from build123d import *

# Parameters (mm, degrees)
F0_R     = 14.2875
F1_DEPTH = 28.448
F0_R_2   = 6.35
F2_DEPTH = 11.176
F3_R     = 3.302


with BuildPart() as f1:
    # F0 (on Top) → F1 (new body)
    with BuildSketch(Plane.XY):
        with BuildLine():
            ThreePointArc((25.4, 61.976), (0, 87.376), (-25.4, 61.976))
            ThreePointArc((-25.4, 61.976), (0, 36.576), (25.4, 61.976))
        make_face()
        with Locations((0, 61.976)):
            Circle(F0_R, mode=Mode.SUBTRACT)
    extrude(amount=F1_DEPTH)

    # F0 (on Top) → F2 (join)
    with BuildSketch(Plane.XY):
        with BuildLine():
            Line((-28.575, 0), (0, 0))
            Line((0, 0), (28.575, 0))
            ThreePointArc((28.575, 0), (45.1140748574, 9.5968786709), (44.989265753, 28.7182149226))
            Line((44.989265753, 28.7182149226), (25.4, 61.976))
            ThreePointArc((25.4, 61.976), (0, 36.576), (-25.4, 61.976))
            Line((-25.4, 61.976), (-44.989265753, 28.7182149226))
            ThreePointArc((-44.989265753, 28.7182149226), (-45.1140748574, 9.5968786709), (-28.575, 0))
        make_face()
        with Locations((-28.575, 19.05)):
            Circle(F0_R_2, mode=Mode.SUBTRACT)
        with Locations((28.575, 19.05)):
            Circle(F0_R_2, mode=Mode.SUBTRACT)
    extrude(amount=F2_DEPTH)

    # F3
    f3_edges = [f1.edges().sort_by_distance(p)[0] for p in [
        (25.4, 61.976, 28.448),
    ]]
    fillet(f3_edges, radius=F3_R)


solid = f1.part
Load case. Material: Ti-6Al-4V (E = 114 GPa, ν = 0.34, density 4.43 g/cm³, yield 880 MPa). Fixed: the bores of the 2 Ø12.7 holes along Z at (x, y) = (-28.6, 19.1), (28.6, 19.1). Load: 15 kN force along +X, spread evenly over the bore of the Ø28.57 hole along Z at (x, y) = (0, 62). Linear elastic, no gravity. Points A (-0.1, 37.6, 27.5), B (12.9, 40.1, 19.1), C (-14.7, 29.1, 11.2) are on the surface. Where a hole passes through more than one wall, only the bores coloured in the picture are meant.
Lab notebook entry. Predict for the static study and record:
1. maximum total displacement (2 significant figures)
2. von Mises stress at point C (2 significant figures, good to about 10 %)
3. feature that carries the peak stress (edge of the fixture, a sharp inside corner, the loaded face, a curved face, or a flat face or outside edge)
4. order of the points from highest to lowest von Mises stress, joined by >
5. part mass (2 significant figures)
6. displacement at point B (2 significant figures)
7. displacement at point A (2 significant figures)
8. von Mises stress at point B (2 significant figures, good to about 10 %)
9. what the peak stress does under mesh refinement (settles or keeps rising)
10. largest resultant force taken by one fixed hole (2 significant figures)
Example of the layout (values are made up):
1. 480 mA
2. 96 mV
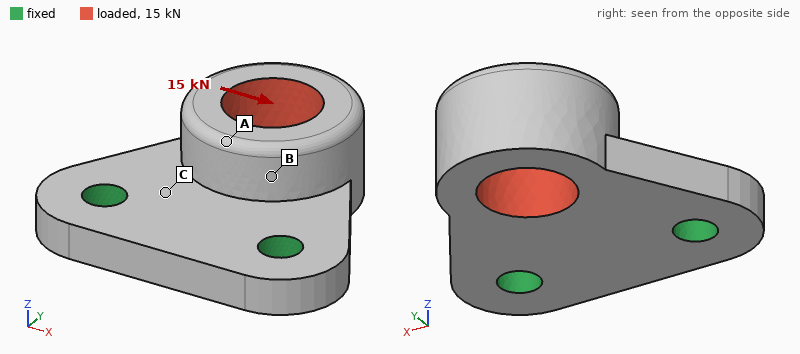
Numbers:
1. 59 µm
2. 45 MPa
3. edge of the fixture
4. C > B > A
5. 350 g
6. 23 µm
7. 28 µm
8. 17 MPa
9. keeps rising
10. 12 kN
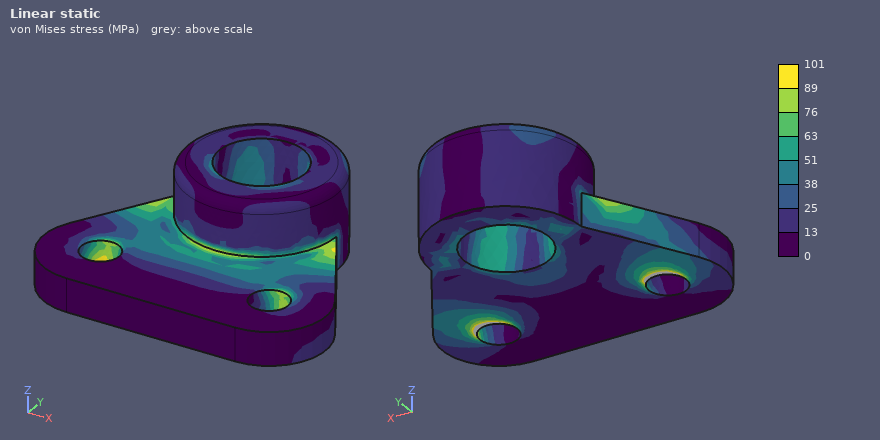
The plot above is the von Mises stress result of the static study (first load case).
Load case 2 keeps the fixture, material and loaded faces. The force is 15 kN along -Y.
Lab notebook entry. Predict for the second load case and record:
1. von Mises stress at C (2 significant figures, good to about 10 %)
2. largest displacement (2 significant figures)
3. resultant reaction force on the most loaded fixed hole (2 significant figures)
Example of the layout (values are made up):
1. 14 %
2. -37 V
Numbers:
1. 77 MPa
2. 0.20 mm
3. 7.8 kN
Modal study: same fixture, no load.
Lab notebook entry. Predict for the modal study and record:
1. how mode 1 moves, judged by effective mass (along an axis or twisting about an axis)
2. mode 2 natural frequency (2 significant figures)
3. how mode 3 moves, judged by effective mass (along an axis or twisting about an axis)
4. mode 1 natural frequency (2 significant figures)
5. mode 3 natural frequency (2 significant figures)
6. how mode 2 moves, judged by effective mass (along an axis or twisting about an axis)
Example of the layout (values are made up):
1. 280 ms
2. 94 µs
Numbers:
1. along Z
2. 6400 Hz
3. along X
4. 2100 Hz
5. 8000 Hz
6. along X
